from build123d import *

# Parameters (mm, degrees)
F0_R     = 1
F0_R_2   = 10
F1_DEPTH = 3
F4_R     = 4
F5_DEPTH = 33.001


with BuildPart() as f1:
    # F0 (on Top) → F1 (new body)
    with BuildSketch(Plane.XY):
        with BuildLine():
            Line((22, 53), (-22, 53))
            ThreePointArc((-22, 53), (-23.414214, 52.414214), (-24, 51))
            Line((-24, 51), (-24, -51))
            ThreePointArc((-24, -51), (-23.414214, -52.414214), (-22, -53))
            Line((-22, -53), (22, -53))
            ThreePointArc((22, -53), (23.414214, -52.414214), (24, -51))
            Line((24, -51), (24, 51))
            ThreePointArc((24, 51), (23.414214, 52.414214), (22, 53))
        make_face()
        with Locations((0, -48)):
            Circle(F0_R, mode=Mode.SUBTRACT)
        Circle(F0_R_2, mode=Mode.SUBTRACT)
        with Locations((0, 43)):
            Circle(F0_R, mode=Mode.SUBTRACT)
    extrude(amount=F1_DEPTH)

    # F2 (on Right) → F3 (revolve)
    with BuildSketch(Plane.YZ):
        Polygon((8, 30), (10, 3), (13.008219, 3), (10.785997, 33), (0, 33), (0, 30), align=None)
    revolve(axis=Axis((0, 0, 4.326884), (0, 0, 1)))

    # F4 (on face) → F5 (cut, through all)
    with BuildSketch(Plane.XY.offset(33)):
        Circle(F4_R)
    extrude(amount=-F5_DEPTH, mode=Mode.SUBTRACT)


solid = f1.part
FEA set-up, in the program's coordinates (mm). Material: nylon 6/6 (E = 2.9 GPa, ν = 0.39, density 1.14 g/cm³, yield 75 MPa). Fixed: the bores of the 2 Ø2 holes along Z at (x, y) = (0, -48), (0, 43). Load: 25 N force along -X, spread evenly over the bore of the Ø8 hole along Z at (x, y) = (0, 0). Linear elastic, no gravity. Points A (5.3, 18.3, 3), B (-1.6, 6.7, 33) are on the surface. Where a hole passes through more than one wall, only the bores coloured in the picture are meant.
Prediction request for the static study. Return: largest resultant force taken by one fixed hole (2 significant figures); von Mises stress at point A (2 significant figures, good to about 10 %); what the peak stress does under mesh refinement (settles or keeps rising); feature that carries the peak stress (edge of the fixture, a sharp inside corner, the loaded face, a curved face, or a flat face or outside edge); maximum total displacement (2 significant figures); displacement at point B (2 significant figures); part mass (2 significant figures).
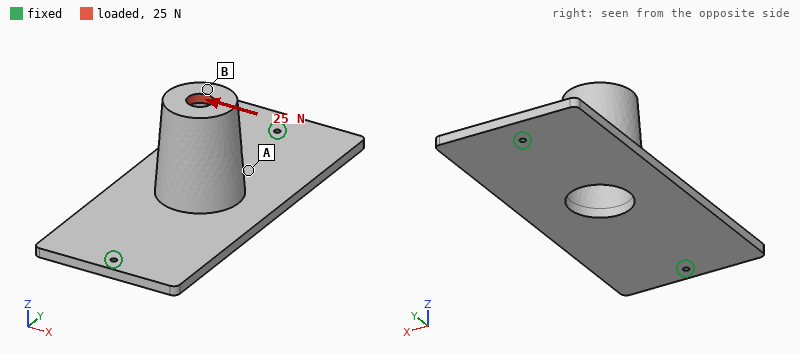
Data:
13 N
4.1 MPa
keeps rising
edge of the fixture
1.3 mm
1.2 mm
24 g
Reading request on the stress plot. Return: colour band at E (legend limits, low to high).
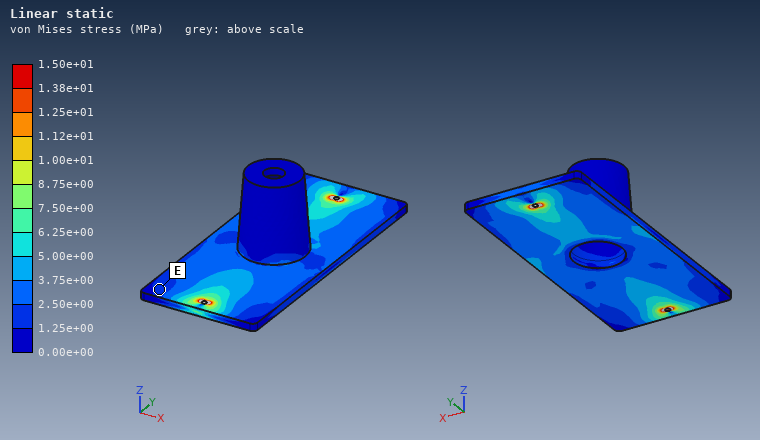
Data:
1.25e+00 to 2.50e+00 MPa
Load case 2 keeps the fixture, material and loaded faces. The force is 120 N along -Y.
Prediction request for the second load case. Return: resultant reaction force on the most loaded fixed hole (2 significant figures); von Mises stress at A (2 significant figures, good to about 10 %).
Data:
81 N
13 MPa
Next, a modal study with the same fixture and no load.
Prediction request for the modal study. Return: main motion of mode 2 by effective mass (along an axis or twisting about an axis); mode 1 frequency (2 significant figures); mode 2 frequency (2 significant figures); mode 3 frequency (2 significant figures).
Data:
along Z
320 Hz
400 Hz
760 Hz
